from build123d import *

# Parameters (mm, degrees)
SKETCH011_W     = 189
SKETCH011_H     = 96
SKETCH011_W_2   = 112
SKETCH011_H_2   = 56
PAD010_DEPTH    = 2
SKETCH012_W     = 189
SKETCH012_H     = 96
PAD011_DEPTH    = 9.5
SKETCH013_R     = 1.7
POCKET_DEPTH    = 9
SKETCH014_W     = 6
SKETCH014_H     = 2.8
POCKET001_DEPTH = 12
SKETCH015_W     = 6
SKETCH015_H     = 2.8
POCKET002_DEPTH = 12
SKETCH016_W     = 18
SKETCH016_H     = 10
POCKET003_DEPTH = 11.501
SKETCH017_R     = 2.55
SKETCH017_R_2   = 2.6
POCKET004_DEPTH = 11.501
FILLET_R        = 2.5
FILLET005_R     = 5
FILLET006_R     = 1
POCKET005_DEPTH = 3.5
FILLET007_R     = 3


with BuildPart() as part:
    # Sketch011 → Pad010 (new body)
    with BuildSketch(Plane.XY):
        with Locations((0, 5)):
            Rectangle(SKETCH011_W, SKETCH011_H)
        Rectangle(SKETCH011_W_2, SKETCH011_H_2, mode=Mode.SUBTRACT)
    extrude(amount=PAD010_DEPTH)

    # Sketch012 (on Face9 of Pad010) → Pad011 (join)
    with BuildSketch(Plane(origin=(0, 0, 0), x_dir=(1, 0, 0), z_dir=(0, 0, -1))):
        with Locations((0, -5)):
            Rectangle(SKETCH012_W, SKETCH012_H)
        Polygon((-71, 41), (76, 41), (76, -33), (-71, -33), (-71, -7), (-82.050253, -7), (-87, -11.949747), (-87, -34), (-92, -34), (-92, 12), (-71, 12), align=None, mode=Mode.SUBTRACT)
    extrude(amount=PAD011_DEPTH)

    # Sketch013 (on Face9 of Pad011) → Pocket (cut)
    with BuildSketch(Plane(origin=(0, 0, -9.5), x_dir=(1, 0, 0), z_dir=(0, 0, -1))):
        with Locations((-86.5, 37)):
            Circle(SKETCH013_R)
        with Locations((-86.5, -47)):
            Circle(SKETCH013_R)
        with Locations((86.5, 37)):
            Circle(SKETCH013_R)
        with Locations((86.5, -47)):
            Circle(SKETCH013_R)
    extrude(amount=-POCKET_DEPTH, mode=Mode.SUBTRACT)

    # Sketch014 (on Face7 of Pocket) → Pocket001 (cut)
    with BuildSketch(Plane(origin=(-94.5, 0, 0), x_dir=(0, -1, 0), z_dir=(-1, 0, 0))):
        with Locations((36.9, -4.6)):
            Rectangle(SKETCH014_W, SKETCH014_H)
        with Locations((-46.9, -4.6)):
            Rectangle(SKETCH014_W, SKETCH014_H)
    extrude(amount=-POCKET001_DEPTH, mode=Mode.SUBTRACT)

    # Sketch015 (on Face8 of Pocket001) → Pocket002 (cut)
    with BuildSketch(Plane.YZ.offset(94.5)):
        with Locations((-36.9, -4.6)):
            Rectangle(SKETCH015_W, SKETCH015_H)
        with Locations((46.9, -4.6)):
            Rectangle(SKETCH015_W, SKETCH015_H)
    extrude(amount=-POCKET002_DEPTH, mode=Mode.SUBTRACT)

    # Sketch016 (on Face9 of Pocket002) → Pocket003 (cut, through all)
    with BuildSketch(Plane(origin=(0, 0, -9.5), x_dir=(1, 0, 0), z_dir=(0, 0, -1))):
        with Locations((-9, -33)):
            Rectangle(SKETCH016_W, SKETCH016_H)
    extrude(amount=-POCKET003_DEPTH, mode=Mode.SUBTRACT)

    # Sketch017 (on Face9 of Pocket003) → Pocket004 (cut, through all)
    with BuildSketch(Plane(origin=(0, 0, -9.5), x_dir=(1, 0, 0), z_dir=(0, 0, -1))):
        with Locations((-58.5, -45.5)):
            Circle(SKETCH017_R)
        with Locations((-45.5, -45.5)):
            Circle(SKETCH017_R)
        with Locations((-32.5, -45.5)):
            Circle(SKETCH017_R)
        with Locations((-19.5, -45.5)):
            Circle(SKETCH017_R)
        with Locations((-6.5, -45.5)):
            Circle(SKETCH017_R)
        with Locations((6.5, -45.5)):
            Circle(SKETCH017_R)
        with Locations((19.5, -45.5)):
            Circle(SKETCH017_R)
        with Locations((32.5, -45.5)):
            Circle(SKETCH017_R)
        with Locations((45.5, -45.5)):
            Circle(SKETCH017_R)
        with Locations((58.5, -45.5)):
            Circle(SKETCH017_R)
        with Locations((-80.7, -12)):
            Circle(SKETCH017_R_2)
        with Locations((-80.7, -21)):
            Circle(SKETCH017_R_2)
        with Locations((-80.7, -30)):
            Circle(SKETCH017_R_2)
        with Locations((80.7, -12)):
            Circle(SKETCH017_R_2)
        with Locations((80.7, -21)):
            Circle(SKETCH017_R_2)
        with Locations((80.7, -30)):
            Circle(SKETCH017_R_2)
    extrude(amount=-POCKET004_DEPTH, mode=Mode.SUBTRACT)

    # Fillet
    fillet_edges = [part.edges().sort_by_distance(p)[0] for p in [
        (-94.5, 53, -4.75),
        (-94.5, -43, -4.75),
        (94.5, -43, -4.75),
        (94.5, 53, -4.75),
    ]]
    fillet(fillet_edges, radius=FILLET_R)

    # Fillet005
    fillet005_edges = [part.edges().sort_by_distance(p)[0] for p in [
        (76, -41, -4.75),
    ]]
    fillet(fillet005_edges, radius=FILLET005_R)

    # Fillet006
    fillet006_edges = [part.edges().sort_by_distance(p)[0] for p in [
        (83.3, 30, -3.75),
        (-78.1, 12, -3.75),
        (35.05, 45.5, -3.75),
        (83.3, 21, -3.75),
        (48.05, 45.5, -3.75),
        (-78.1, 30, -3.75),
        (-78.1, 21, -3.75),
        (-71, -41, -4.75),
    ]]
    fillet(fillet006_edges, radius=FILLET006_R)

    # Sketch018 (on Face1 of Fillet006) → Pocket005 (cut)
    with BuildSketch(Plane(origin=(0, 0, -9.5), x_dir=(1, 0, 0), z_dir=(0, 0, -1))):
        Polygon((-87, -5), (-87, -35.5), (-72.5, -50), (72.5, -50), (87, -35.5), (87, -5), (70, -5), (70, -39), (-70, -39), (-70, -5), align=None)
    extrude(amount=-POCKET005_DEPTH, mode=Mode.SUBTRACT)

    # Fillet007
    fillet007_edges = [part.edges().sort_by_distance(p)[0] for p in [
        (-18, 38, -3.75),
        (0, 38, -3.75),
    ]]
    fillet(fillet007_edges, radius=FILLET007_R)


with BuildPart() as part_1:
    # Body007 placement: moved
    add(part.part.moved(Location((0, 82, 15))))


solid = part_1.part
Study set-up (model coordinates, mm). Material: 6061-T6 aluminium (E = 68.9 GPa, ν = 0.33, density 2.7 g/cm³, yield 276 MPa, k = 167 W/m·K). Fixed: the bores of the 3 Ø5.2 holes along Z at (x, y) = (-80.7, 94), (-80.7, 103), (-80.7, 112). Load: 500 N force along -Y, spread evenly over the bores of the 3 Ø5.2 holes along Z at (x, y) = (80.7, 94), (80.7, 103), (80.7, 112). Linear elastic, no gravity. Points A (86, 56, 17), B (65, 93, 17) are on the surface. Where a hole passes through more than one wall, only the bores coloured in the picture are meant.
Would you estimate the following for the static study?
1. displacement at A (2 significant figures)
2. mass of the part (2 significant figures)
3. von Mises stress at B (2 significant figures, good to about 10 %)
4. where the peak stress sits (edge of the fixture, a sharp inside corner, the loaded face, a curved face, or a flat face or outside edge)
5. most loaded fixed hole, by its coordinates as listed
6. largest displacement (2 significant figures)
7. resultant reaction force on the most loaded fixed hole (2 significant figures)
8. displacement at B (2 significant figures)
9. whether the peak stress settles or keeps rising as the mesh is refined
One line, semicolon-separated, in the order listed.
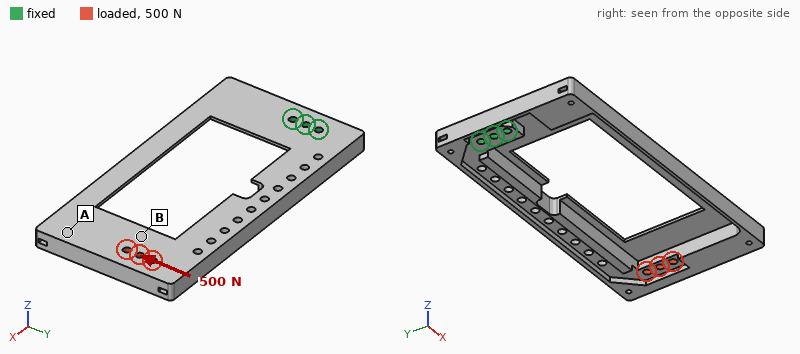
0.54 mm; 200 g; 17 MPa; edge of the fixture; (-80.7, 112); 0.69 mm; 3.3 kN; 0.52 mm; keeps rising
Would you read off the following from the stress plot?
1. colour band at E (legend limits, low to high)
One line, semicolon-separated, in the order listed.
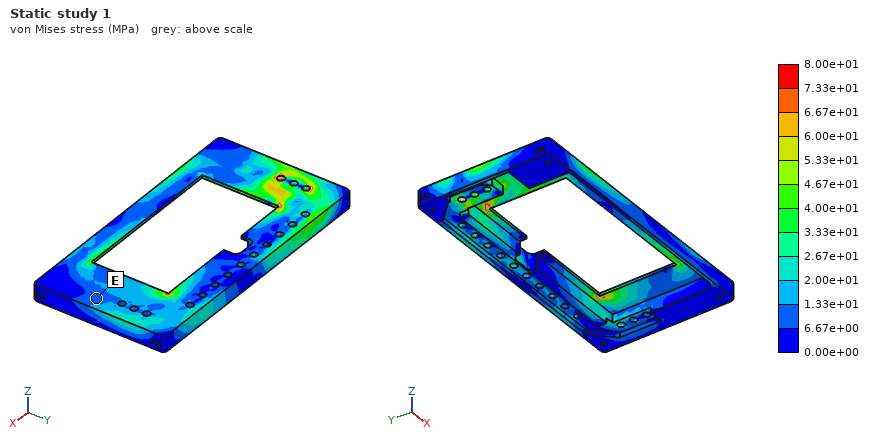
6.67e+00 to 1.33e+01 MPa
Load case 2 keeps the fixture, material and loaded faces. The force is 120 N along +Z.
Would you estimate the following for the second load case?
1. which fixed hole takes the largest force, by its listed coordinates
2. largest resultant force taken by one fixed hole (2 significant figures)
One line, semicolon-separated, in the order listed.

(-80.7, 103); 270 N
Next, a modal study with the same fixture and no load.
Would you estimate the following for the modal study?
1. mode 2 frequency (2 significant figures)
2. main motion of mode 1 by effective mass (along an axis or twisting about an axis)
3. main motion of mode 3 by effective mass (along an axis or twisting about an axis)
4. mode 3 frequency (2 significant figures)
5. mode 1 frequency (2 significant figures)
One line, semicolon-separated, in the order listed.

400 Hz; along Z; along Y; 550 Hz; 150 Hz
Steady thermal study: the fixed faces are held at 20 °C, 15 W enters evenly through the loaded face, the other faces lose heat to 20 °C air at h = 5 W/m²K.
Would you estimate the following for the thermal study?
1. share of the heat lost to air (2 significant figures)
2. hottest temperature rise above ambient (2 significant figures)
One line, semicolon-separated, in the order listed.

32 %; 54 K
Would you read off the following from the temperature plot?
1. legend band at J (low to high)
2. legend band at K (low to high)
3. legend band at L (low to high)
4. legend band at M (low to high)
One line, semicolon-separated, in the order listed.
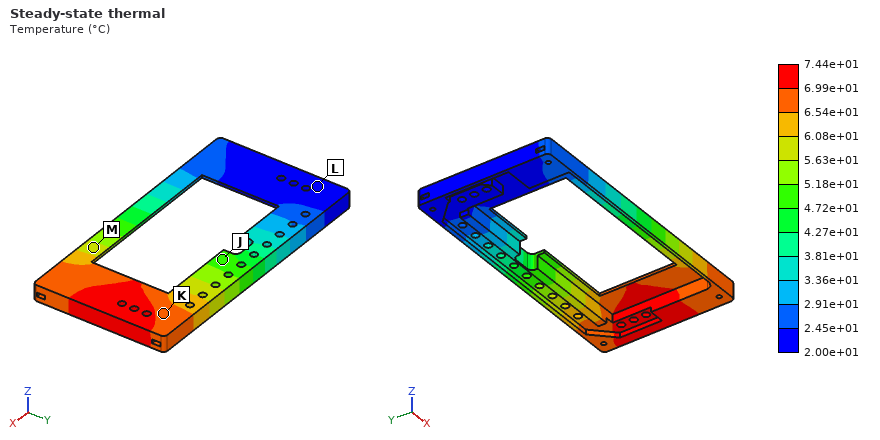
4.72e+01 to 5.18e+01 °C; 6.54e+01 to 6.99e+01 °C; 2.00e+01 to 2.45e+01 °C; 5.63e+01 to 6.08e+01 °C
